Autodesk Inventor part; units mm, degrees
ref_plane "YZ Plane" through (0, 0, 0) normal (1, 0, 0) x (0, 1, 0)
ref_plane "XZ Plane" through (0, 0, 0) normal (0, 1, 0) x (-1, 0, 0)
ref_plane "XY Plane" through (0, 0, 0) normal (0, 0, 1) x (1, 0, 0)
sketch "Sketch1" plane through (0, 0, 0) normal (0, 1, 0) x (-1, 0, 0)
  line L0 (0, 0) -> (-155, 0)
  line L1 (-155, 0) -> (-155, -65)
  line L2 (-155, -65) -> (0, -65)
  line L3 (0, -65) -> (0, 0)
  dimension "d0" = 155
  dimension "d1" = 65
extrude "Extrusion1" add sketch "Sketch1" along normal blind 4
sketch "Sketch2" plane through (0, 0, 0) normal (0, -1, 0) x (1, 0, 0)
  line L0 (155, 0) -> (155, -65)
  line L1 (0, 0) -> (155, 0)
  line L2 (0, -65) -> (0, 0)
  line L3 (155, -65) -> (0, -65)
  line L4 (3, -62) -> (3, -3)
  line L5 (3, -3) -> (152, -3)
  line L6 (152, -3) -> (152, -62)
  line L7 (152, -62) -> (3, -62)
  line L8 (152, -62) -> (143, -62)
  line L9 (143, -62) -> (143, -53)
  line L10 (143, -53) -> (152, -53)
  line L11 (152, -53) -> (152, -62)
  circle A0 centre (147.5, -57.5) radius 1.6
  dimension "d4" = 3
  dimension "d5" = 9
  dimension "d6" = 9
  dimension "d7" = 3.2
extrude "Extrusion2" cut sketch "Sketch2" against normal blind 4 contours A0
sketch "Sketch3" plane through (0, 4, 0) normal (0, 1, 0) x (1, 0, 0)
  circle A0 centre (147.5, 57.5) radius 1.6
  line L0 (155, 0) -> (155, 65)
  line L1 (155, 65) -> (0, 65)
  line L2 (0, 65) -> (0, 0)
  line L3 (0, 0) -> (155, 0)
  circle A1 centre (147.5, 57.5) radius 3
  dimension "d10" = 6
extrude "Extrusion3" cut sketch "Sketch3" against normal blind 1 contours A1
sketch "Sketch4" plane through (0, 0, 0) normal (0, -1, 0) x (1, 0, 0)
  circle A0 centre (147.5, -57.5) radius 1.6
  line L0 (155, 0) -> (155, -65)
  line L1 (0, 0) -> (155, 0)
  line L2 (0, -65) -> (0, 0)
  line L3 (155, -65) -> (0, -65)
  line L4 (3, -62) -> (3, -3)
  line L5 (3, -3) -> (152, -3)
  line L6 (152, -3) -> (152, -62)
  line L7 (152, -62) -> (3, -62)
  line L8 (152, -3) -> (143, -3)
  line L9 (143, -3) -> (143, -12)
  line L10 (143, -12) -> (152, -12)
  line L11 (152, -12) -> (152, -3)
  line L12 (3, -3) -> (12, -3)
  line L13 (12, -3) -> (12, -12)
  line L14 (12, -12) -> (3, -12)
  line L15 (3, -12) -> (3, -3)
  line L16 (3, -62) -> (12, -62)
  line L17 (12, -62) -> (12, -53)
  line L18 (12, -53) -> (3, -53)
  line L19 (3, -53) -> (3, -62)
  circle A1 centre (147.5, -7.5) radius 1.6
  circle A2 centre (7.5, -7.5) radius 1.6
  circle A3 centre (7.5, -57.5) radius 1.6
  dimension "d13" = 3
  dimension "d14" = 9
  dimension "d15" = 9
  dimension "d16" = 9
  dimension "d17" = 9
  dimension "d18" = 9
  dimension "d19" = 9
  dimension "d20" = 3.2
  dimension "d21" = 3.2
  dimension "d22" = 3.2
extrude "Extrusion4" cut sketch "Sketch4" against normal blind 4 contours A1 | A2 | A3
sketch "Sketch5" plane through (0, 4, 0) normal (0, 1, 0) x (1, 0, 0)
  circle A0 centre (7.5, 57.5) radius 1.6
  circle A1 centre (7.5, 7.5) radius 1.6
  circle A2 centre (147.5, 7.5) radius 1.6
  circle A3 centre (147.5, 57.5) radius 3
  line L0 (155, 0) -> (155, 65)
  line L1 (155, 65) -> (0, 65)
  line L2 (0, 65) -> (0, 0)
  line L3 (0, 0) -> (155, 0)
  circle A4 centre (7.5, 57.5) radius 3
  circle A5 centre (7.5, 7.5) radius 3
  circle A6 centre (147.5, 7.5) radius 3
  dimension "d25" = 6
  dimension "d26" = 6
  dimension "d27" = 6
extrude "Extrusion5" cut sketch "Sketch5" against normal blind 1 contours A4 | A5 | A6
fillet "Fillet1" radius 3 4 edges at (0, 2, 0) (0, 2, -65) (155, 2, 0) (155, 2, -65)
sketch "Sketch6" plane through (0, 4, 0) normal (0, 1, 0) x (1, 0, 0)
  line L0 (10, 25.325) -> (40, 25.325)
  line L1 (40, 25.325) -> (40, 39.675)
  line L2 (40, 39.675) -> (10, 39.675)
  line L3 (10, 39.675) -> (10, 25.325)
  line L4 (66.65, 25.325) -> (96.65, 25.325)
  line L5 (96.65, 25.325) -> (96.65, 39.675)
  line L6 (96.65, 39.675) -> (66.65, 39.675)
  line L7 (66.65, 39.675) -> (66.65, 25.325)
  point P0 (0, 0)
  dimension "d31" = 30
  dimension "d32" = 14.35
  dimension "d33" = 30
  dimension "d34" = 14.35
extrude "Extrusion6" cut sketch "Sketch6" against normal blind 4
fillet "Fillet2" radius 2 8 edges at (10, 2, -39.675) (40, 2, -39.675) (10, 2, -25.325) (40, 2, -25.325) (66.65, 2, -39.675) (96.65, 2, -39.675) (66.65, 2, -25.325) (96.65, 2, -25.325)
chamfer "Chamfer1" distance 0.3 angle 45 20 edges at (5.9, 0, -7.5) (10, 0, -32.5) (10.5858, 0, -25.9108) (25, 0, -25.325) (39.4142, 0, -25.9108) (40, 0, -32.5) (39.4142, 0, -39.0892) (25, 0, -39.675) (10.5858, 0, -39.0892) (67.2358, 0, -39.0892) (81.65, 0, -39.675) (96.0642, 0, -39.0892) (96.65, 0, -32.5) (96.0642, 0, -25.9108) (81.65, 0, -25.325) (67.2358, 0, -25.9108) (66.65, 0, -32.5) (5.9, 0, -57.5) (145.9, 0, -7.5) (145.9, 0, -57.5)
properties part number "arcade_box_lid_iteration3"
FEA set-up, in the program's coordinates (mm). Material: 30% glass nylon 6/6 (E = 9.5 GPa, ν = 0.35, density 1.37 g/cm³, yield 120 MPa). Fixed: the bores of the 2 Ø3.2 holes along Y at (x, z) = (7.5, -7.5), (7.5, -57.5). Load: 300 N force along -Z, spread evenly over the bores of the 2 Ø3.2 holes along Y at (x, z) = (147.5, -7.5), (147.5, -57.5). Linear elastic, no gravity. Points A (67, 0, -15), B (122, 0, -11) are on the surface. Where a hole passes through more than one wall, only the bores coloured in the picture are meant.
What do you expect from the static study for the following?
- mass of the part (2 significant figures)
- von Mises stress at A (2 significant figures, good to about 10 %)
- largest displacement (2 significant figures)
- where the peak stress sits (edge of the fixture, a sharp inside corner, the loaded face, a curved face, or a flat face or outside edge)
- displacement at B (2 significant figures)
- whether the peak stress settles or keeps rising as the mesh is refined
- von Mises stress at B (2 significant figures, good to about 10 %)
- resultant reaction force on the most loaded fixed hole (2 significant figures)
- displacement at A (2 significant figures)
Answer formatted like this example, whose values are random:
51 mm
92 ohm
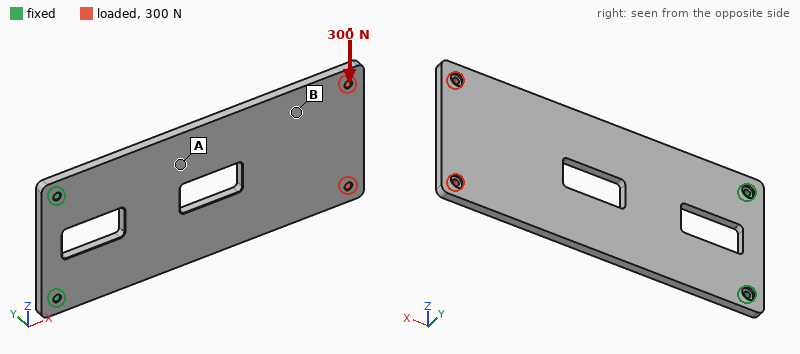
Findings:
50 g
6.2 MPa
0.54 mm
edge of the fixture
0.39 mm
keeps rising
2.7 MPa
840 N
0.16 mm
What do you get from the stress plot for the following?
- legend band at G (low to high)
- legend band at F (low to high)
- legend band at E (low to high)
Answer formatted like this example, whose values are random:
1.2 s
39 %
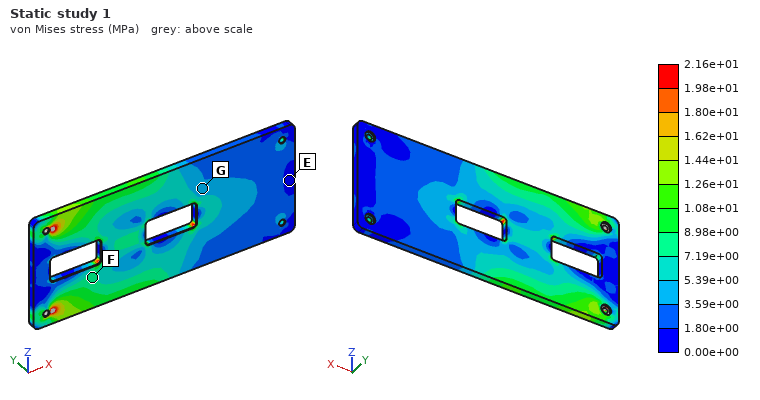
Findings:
3.59e+00 to 5.39e+00 MPa
7.19e+00 to 8.98e+00 MPa
0.00e+00 to 1.80e+00 MPa
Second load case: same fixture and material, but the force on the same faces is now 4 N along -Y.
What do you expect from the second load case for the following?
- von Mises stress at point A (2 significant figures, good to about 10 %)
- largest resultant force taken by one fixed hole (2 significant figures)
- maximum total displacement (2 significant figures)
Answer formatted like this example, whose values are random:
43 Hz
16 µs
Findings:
2.3 MPa
2.1 N
1.7 mm
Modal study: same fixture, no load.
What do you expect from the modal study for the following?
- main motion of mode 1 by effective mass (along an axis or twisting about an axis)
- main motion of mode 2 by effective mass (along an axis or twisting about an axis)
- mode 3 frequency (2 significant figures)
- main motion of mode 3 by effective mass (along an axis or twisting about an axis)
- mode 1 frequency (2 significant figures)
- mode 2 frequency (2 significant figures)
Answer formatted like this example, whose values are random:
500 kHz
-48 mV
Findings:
along Y
twisting about X
440 Hz
along Y
66 Hz
340 Hz
